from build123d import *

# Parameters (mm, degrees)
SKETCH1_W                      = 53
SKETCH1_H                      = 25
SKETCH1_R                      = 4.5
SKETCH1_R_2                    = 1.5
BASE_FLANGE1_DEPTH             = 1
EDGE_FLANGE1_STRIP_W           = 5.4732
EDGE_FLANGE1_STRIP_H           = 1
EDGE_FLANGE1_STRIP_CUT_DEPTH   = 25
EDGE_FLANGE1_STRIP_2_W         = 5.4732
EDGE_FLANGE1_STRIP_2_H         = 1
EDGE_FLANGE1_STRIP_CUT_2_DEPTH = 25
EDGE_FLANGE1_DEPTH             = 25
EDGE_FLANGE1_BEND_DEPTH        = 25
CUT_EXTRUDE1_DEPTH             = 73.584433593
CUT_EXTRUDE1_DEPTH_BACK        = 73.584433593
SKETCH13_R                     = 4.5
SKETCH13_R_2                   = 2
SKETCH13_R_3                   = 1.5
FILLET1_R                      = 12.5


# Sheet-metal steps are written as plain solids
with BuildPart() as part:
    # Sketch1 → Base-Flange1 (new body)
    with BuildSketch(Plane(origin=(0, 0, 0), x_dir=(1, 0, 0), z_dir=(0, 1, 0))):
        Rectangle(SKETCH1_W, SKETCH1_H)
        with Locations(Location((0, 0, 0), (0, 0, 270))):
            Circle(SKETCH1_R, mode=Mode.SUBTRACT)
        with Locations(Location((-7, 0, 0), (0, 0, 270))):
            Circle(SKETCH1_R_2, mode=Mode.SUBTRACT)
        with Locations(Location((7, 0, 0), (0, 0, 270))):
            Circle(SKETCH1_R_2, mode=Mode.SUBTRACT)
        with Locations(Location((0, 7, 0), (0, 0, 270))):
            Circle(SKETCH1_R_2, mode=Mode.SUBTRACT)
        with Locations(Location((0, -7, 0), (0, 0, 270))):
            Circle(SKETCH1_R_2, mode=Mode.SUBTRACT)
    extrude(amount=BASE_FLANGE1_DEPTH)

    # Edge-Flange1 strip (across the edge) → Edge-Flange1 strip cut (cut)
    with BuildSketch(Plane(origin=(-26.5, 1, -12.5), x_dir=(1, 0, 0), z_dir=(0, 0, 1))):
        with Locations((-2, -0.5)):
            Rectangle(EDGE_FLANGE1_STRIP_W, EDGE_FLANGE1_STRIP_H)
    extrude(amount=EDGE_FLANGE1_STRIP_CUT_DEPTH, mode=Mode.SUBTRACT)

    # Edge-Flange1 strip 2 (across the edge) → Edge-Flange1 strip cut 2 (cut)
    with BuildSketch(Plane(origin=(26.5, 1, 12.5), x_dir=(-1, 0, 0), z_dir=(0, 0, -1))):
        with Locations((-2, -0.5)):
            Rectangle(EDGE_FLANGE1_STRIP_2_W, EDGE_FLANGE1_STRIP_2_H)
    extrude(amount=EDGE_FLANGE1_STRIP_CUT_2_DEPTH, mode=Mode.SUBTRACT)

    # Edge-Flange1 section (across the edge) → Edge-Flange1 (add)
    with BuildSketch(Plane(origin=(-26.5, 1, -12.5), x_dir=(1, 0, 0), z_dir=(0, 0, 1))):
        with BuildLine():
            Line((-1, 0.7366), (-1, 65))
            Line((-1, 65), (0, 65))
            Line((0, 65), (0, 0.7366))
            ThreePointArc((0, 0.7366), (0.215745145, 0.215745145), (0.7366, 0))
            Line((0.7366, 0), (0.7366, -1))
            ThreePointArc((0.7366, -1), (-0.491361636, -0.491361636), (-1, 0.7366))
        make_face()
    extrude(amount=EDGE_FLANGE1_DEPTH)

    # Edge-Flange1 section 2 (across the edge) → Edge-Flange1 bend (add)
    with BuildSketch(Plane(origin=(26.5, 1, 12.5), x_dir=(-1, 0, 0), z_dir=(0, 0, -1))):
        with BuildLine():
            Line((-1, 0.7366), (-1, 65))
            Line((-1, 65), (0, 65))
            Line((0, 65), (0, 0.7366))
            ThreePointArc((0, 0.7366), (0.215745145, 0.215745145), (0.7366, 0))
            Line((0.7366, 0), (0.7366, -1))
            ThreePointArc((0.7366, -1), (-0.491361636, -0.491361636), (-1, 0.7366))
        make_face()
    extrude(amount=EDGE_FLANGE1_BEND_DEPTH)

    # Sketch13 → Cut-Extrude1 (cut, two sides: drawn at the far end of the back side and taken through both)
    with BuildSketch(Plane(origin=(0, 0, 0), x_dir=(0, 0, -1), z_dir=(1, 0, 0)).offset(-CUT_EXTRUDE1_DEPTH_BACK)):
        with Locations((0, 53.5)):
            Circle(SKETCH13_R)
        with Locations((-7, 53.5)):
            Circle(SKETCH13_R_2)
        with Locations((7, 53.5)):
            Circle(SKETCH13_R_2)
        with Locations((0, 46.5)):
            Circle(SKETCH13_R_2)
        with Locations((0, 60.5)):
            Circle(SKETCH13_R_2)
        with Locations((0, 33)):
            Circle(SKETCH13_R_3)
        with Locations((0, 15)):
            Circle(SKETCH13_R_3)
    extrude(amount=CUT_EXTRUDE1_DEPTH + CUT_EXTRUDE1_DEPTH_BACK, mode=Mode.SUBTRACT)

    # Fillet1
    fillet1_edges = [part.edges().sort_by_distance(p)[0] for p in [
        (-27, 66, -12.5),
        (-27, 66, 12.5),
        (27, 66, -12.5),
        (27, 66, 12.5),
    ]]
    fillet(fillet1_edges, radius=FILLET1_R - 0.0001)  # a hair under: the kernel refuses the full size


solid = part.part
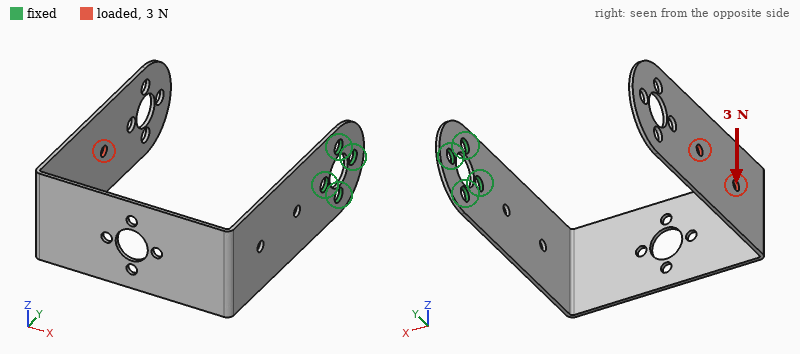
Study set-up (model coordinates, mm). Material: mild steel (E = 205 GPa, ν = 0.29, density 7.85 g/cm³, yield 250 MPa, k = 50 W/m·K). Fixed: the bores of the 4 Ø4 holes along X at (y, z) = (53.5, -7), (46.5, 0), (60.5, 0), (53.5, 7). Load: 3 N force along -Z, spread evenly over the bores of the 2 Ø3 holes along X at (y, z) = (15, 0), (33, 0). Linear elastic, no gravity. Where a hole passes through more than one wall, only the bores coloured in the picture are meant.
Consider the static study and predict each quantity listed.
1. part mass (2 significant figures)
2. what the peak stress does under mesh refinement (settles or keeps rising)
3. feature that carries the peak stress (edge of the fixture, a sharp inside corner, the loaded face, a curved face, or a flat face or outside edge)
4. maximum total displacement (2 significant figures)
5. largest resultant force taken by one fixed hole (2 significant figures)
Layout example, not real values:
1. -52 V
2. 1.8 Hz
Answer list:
1. 32 g
2. keeps rising
3. edge of the fixture
4. 1.0 mm
5. 3.8 N
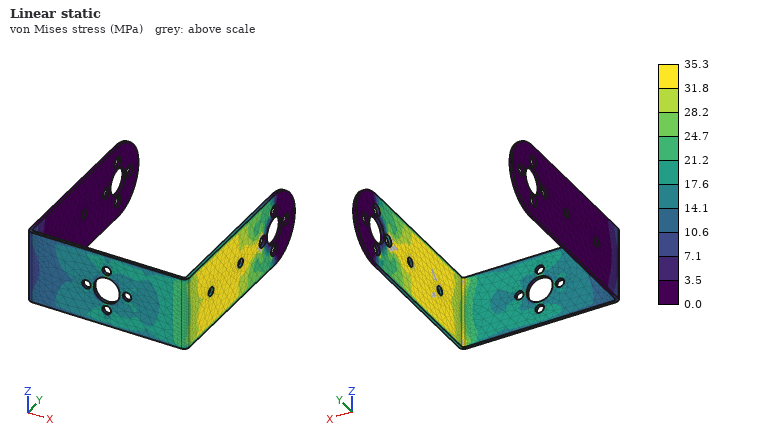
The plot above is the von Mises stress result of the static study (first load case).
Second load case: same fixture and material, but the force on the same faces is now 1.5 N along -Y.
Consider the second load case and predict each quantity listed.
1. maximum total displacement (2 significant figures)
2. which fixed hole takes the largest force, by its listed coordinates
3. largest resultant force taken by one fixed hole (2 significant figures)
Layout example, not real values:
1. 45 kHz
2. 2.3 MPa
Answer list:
1. 1.00 mm
2. (46.5, 0)
3. 5.9 N
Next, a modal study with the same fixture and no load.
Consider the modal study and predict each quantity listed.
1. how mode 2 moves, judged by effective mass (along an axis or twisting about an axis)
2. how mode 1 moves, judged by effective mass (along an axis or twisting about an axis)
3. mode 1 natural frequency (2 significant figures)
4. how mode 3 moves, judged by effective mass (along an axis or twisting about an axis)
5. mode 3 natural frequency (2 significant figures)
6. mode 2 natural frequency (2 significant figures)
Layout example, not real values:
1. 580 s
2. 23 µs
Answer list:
1. along Z
2. along Y
3. 56 Hz
4. along X
5. 120 Hz
6. 82 Hz
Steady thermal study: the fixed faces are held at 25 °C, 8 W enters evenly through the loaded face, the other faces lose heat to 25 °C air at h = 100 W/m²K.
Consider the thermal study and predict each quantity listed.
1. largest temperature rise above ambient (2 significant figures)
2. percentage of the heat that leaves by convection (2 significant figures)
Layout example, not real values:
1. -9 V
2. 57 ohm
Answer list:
1. 49 K
2. 100 %
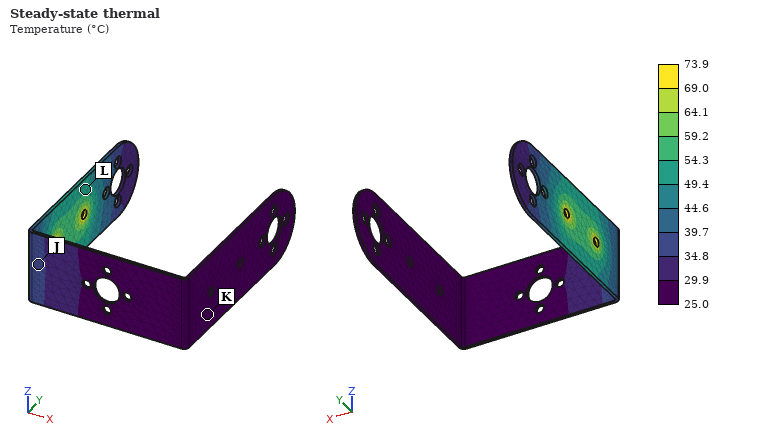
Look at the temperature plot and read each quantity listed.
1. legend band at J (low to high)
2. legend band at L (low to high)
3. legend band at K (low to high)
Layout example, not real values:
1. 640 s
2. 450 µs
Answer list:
1. 34.8 to 39.7 °C
2. 49.4 to 54.3 °C
3. 25.0 to 29.9 °C
